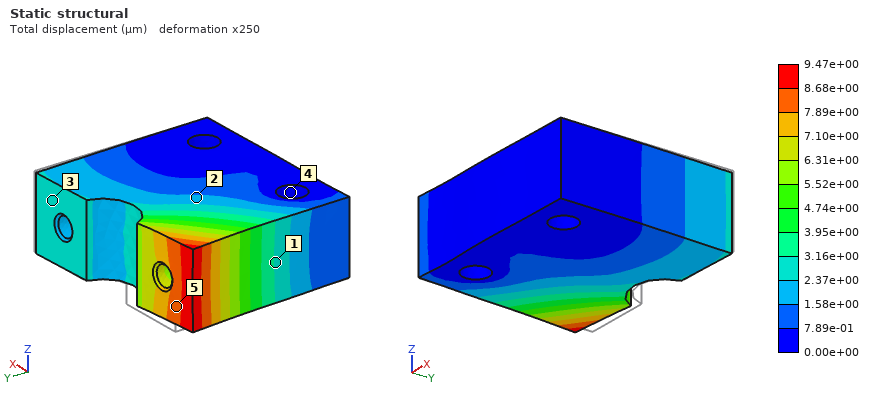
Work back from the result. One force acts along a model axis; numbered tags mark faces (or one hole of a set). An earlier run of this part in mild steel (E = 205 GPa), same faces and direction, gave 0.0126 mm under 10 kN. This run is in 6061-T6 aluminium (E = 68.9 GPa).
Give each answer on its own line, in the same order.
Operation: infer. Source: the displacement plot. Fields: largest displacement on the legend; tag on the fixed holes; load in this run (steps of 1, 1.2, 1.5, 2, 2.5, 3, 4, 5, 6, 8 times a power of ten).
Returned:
9.47e+00 µm
4
2.5 kN
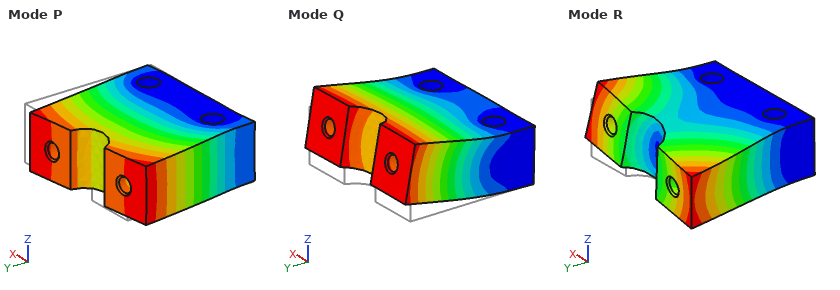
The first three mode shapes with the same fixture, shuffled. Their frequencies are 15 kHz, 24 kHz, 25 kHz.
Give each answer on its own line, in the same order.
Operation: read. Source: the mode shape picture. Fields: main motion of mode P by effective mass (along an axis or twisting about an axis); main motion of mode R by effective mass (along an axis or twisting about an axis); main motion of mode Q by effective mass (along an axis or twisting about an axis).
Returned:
along X
twisting about Y
along Z
